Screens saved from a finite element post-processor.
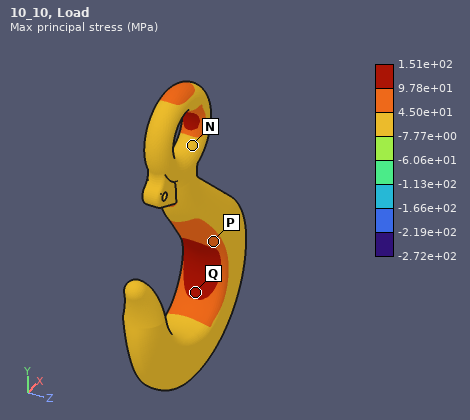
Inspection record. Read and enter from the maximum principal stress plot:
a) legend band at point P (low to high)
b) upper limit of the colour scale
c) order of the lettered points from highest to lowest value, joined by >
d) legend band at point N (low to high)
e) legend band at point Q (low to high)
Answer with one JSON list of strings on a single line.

["4.50e+01 to 9.78e+01 MPa", "1.51e+02 MPa", "Q > P > N", "-7.77e+00 to 4.50e+01 MPa", "9.78e+01 to 1.51e+02 MPa"]
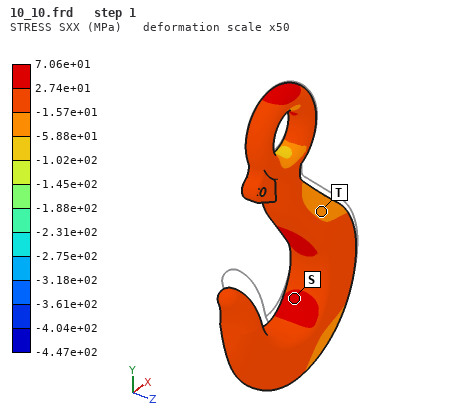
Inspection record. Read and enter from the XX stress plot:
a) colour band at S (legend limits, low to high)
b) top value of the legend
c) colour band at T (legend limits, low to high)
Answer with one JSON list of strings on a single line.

["2.74e+01 to 7.06e+01 MPa", "7.06e+01 MPa", "-5.88e+01 to -1.57e+01 MPa"]
